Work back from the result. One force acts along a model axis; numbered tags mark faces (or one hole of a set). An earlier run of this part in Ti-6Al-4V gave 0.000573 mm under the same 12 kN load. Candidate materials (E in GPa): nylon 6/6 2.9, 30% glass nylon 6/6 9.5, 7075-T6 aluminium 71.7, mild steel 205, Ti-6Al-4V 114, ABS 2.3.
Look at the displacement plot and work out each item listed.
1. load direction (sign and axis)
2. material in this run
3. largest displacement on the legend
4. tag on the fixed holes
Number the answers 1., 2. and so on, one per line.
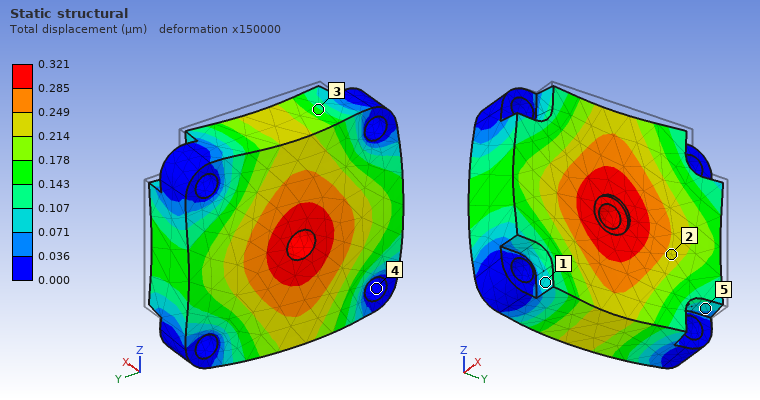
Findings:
1. -X
2. mild steel
3. 0.321 µm
4. 4
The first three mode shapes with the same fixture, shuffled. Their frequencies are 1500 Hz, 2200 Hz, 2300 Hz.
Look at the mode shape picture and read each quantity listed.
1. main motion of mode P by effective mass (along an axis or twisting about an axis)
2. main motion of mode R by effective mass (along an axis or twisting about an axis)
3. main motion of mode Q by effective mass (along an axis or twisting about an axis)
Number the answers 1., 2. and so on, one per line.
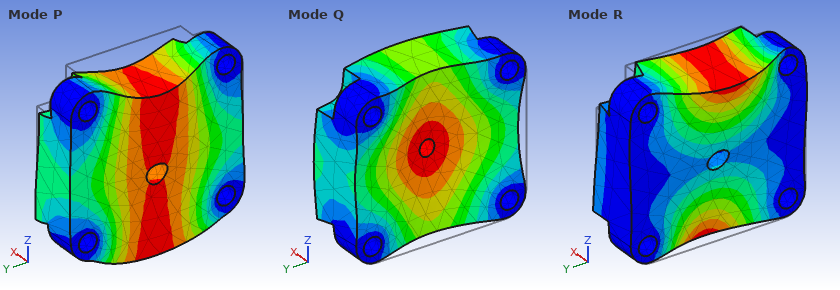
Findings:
1. along Z
2. twisting about Y
3. along X
